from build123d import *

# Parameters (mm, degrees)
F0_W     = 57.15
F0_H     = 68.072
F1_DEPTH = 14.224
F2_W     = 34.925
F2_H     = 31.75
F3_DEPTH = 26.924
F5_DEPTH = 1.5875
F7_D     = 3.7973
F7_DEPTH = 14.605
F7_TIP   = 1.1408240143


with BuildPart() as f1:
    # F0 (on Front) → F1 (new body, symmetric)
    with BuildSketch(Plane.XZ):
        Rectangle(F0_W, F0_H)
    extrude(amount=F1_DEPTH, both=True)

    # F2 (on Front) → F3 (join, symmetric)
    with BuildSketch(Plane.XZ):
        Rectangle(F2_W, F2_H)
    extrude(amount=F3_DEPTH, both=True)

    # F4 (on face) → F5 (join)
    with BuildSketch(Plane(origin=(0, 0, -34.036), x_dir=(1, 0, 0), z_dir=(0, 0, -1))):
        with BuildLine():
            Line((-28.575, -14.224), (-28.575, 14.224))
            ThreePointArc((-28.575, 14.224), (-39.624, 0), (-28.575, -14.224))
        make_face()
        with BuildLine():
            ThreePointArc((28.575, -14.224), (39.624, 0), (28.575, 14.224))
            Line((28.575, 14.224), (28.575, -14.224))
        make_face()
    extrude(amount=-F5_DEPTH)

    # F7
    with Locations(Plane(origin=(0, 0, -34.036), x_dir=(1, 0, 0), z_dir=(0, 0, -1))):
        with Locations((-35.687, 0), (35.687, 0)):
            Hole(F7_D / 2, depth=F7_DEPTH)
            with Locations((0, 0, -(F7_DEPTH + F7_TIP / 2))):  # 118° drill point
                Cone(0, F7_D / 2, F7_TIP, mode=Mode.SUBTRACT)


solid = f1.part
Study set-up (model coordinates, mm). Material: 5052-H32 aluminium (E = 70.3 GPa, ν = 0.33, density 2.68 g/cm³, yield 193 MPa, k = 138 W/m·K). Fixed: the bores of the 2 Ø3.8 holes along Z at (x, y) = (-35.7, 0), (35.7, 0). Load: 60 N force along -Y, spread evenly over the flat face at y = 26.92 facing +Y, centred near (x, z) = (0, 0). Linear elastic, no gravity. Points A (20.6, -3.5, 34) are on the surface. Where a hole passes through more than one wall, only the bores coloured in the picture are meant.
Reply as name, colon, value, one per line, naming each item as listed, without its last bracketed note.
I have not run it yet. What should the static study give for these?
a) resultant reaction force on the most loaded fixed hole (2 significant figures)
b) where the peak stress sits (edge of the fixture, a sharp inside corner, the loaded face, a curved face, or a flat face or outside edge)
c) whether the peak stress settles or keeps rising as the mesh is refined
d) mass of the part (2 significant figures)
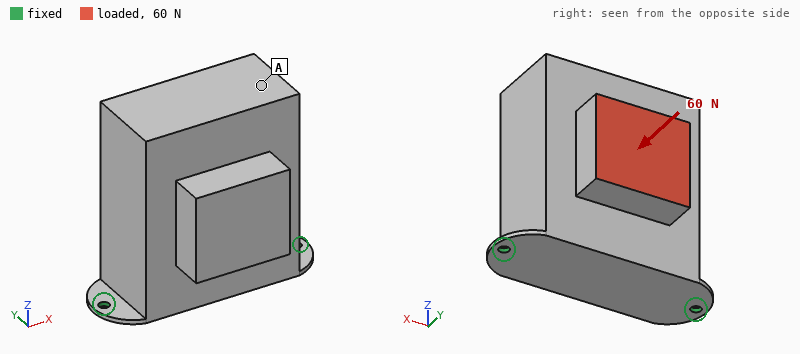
resultant reaction force on the most loaded fixed hole: 30 N
where the peak stress sits: edge of the fixture
whether the peak stress settles or keeps rising as the mesh is refined: keeps rising
mass of the part: 370 g
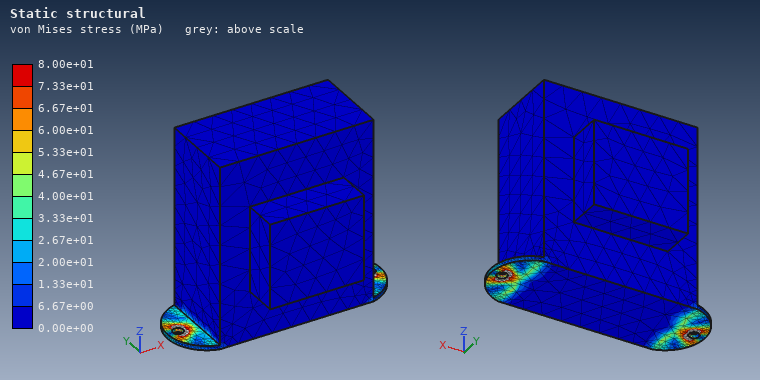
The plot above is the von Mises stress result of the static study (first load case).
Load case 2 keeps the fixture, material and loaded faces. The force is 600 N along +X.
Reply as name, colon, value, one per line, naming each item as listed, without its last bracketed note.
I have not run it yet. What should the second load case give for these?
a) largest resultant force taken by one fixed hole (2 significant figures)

largest resultant force taken by one fixed hole: 490 N
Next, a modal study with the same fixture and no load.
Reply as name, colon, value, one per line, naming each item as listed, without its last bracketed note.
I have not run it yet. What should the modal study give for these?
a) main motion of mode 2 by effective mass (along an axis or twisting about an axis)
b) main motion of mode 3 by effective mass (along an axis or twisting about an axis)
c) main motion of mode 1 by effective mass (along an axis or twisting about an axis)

main motion of mode 2 by effective mass: along X
main motion of mode 3 by effective mass: along Z
main motion of mode 1 by effective mass: along Y
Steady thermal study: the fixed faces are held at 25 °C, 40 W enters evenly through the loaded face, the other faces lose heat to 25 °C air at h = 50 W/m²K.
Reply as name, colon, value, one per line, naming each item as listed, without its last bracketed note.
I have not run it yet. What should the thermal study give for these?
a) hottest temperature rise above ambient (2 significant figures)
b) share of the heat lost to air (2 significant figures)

hottest temperature rise above ambient: 30 K
share of the heat lost to air: 53 %
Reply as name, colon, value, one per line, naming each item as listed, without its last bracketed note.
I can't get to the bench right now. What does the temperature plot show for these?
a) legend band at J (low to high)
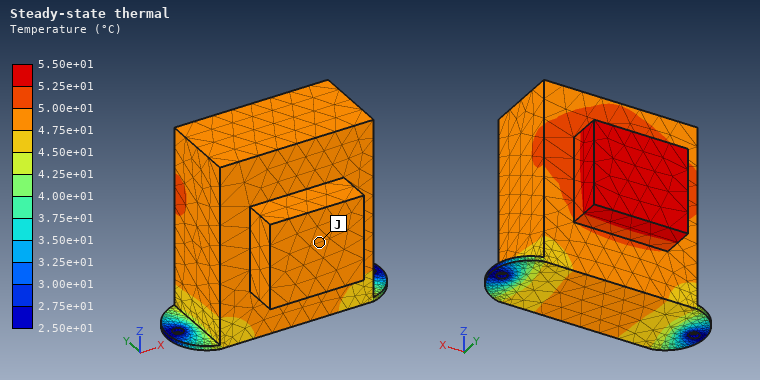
legend band at J: 4.75e+01 to 5.00e+01 °C
